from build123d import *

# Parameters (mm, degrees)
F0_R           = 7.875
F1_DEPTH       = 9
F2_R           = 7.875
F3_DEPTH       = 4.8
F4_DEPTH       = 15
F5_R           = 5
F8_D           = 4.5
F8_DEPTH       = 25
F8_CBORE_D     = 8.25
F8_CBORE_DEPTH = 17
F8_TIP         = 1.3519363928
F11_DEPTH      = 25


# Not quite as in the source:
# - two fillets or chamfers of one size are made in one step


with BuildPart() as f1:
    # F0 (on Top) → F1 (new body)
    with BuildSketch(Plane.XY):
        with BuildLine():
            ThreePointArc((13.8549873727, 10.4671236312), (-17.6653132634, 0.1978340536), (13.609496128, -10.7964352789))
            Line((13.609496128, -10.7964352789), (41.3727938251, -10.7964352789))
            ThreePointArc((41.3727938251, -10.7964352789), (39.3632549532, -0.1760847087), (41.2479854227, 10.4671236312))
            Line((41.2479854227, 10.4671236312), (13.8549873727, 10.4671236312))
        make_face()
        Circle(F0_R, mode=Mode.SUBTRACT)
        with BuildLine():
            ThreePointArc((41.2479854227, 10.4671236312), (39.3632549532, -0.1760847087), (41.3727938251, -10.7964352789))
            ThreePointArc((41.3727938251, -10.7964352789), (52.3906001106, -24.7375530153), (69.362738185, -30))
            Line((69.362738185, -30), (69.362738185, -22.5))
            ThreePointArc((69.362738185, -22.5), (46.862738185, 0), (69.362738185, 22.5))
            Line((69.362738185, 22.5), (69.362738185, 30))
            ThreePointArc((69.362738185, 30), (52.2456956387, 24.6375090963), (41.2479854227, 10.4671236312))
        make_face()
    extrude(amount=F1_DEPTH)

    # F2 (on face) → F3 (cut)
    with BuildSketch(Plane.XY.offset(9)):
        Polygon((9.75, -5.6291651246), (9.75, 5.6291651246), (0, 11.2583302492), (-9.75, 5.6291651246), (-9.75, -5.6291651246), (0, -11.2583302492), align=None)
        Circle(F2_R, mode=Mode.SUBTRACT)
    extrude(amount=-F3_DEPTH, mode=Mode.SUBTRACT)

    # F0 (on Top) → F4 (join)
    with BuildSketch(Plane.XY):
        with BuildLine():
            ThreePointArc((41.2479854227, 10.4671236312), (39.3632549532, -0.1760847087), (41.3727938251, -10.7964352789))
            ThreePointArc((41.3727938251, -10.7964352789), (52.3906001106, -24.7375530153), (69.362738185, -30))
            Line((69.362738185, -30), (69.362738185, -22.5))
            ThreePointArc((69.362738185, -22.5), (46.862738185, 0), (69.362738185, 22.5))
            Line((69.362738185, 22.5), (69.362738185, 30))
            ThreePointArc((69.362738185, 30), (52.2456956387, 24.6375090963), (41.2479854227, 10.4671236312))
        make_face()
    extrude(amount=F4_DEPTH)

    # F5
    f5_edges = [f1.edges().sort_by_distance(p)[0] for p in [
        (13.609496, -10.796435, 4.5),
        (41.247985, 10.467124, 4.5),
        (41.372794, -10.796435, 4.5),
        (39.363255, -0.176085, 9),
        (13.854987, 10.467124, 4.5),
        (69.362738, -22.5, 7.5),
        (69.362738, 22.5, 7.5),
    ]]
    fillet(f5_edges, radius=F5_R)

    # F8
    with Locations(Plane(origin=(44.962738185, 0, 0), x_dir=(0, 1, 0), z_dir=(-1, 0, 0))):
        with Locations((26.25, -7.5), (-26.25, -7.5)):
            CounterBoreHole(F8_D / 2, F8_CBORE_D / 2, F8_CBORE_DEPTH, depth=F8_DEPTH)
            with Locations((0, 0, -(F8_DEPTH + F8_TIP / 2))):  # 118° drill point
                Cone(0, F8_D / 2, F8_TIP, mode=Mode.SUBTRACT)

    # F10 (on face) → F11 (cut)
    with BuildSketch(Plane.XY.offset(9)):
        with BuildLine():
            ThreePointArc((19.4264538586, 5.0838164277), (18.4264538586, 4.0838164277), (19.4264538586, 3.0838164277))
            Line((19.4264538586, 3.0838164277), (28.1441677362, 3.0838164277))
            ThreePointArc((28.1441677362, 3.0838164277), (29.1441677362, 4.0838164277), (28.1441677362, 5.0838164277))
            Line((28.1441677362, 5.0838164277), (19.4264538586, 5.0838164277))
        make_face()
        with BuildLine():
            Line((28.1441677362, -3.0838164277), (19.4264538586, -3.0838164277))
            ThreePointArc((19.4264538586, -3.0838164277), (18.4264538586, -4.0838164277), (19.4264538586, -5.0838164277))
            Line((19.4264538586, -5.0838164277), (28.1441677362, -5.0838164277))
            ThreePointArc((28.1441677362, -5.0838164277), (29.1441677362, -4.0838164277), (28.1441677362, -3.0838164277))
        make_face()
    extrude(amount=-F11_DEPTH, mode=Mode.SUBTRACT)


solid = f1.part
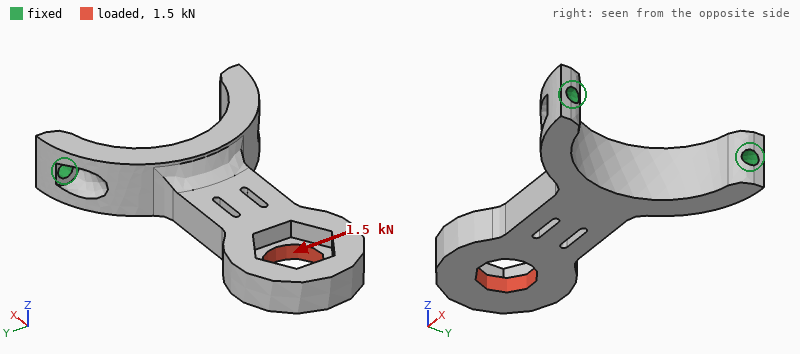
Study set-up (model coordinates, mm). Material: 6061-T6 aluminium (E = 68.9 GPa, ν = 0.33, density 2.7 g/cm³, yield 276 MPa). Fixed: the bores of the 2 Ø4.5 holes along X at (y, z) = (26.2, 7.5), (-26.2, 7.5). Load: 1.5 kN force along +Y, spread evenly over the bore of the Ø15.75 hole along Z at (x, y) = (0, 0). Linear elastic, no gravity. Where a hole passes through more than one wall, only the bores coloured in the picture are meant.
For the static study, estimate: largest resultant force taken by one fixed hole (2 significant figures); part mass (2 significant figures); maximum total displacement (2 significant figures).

2.1 kN
51 g
0.30 mm
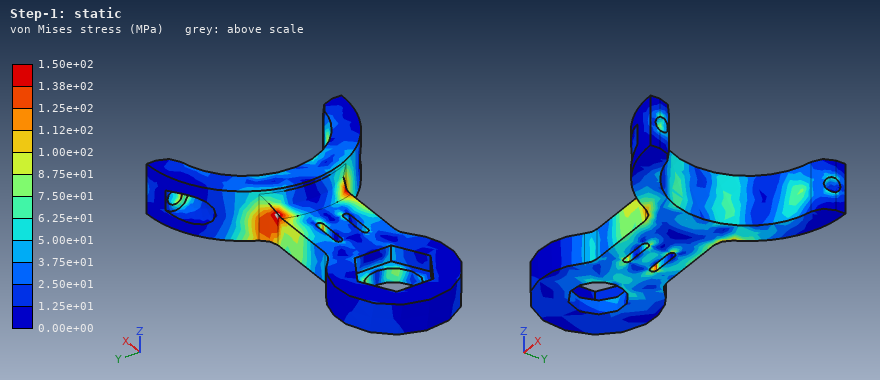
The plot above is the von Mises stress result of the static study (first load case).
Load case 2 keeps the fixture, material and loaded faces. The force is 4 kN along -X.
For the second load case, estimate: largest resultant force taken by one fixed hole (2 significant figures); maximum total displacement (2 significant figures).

2.4 kN
0.51 mm
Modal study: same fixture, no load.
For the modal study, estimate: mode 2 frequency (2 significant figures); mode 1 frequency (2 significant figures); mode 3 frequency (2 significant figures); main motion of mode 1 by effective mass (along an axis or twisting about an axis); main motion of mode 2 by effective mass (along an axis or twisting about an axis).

3000 Hz
1200 Hz
4900 Hz
along Z
along Y
